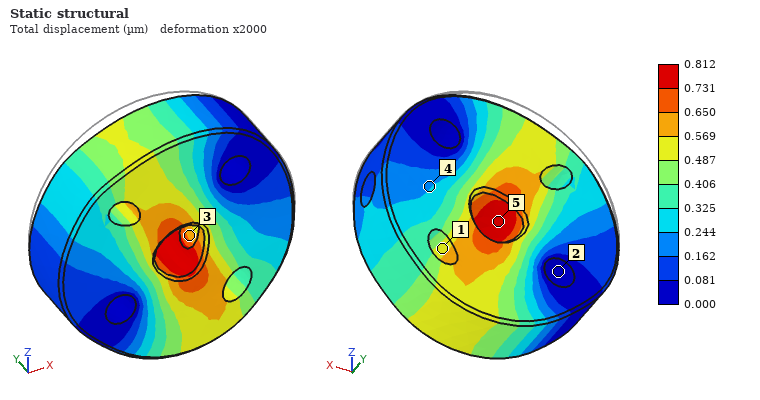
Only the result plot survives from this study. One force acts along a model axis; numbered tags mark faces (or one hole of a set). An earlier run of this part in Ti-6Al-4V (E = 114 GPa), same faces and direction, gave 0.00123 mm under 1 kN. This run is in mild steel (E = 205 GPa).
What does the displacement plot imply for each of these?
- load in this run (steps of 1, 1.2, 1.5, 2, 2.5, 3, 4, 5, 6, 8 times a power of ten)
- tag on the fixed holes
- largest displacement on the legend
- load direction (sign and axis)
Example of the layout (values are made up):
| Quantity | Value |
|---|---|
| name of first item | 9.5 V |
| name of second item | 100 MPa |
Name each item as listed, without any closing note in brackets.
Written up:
| Quantity | Value |
|---|---|
| load in this run | 1.2 kN |
| tag on the fixed holes | 2 |
| largest displacement on the legend | 0.812 µm |
| load direction | -Z |
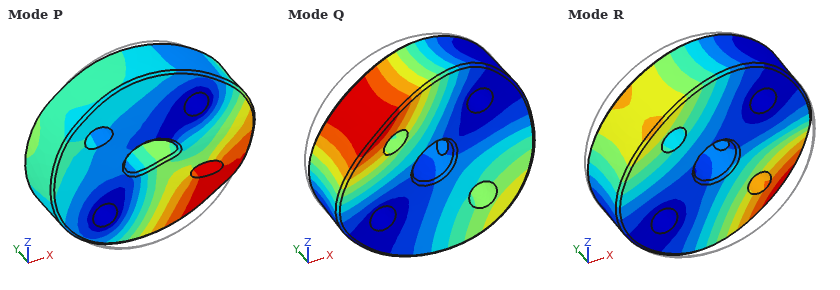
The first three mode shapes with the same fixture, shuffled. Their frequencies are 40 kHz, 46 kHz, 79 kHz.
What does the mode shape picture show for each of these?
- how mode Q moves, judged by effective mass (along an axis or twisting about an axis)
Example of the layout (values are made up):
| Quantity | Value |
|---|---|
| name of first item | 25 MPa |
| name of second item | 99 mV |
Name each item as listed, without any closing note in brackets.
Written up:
| Quantity | Value |
|---|---|
| how mode Q moves, judged by effective mass | along Y |
